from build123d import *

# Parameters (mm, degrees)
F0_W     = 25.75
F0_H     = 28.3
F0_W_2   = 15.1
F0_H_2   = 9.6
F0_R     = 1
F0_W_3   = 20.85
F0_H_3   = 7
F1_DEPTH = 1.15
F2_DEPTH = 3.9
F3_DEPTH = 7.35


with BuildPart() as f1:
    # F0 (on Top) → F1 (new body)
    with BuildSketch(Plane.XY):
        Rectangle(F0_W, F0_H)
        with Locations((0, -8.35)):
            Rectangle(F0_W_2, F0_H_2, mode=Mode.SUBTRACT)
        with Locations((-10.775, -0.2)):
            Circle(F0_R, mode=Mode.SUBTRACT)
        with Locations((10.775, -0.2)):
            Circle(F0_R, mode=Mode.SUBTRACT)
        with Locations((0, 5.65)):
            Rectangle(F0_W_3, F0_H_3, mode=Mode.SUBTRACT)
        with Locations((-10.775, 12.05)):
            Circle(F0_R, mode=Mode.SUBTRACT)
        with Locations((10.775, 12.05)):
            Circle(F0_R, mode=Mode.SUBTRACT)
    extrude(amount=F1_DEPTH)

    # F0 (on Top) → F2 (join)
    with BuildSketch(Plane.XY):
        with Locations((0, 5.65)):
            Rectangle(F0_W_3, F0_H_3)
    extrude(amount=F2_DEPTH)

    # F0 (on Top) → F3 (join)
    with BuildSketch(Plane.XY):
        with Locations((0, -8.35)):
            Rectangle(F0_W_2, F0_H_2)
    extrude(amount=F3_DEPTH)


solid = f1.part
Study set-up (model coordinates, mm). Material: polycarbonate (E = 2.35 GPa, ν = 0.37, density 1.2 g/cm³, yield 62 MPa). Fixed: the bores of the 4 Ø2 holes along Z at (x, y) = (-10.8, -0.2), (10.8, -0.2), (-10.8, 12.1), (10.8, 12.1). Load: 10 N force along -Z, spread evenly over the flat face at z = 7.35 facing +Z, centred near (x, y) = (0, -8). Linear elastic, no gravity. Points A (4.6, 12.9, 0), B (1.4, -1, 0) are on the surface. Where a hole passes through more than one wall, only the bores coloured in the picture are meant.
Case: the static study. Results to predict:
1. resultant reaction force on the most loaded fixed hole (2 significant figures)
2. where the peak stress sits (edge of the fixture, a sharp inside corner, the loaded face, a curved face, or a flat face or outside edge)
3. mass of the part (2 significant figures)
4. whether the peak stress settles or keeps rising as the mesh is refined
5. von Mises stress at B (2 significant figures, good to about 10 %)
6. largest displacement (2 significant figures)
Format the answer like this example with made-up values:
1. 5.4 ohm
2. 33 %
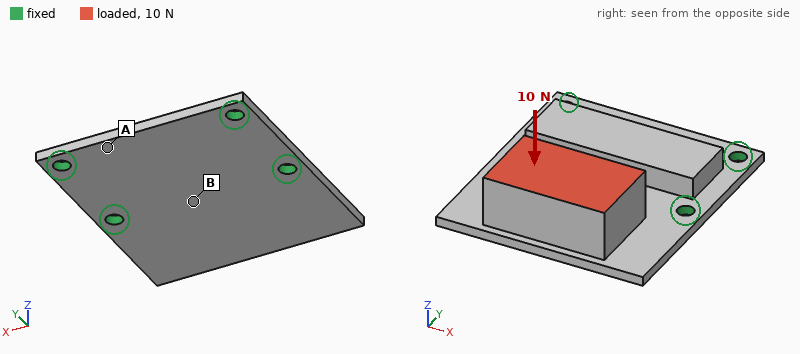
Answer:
1. 6.4 N
2. edge of the fixture
3. 2.5 g
4. keeps rising
5. 6.4 MPa
6. 0.46 mm
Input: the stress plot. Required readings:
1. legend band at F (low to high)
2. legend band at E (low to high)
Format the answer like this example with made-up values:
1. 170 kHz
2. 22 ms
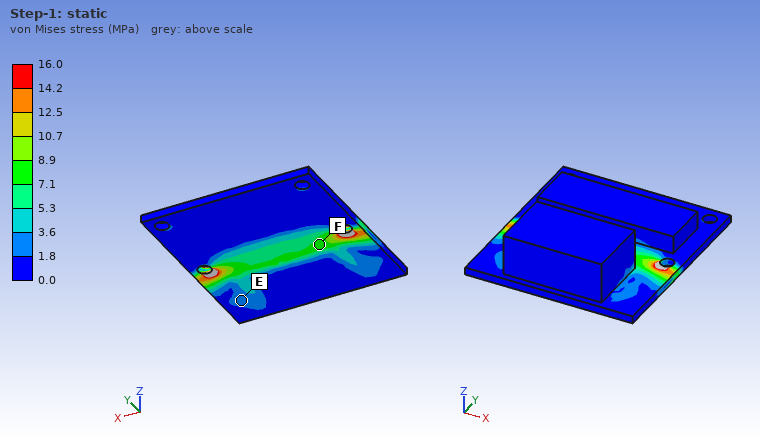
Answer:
1. 7.1 to 8.9 MPa
2. 1.8 to 3.6 MPa
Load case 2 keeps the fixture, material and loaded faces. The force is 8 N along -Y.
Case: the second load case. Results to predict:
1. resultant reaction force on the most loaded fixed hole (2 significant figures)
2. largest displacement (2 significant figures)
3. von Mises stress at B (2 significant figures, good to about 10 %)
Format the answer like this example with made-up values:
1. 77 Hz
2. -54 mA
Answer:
1. 2.8 N
2. 0.38 mm
3. 5.9 MPa
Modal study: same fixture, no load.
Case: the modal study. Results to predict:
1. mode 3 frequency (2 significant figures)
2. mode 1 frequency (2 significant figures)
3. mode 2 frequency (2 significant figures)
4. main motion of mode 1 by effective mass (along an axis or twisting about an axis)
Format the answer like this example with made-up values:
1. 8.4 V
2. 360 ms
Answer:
1. 4000 Hz
2. 710 Hz
3. 3100 Hz
4. along Z
